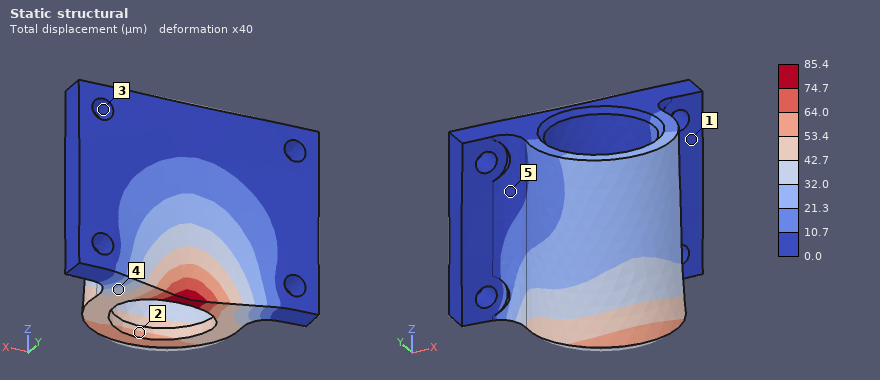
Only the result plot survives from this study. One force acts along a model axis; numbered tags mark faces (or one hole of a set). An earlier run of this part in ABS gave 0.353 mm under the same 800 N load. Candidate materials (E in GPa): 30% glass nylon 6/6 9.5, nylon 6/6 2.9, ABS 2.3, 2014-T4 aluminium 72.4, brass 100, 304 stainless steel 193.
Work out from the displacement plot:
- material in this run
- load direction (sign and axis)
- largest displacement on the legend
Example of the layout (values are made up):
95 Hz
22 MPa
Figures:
30% glass nylon 6/6
-Y
85.4 µm
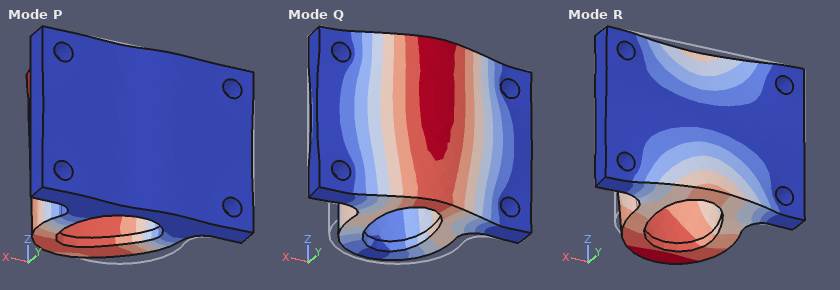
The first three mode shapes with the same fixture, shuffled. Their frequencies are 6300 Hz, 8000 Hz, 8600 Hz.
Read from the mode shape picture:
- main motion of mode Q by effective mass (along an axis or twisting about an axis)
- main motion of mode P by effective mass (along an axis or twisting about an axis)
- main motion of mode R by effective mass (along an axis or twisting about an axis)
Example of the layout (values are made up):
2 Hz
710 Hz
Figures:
along Y
along X
along Z
